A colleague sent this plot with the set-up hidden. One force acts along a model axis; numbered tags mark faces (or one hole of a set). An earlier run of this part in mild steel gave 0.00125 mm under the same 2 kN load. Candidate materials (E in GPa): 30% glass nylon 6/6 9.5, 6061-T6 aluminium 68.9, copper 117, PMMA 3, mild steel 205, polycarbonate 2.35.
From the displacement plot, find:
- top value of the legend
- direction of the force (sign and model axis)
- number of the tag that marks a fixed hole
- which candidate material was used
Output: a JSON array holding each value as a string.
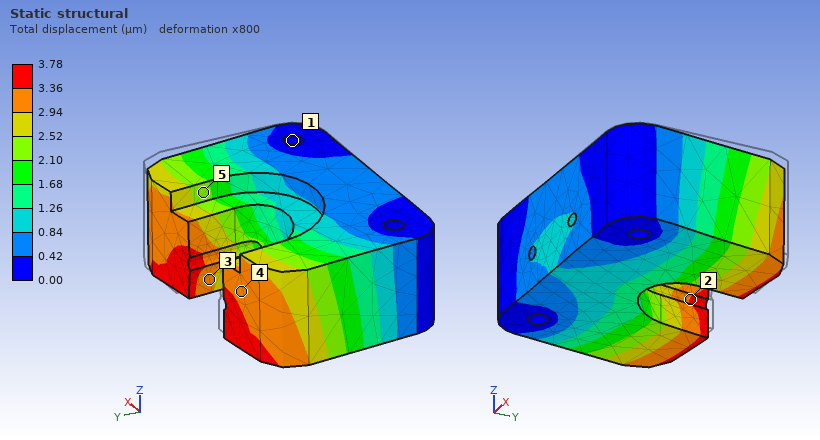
["3.78 µm", "-X", "1", "6061-T6 aluminium"]
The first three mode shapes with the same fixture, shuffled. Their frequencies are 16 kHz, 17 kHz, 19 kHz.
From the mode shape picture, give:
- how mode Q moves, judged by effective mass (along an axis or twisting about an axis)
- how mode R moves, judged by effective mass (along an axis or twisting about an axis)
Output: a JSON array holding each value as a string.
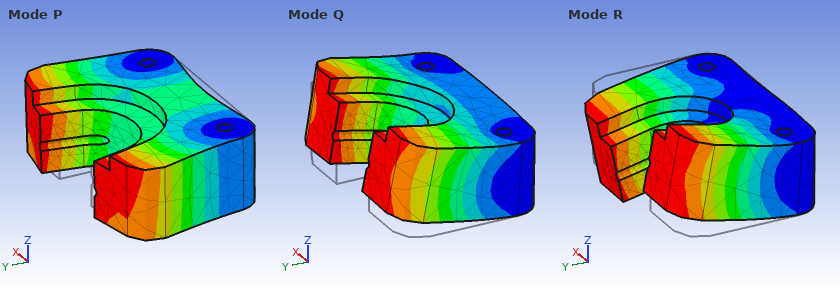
["along Z", "twisting about Y"]
